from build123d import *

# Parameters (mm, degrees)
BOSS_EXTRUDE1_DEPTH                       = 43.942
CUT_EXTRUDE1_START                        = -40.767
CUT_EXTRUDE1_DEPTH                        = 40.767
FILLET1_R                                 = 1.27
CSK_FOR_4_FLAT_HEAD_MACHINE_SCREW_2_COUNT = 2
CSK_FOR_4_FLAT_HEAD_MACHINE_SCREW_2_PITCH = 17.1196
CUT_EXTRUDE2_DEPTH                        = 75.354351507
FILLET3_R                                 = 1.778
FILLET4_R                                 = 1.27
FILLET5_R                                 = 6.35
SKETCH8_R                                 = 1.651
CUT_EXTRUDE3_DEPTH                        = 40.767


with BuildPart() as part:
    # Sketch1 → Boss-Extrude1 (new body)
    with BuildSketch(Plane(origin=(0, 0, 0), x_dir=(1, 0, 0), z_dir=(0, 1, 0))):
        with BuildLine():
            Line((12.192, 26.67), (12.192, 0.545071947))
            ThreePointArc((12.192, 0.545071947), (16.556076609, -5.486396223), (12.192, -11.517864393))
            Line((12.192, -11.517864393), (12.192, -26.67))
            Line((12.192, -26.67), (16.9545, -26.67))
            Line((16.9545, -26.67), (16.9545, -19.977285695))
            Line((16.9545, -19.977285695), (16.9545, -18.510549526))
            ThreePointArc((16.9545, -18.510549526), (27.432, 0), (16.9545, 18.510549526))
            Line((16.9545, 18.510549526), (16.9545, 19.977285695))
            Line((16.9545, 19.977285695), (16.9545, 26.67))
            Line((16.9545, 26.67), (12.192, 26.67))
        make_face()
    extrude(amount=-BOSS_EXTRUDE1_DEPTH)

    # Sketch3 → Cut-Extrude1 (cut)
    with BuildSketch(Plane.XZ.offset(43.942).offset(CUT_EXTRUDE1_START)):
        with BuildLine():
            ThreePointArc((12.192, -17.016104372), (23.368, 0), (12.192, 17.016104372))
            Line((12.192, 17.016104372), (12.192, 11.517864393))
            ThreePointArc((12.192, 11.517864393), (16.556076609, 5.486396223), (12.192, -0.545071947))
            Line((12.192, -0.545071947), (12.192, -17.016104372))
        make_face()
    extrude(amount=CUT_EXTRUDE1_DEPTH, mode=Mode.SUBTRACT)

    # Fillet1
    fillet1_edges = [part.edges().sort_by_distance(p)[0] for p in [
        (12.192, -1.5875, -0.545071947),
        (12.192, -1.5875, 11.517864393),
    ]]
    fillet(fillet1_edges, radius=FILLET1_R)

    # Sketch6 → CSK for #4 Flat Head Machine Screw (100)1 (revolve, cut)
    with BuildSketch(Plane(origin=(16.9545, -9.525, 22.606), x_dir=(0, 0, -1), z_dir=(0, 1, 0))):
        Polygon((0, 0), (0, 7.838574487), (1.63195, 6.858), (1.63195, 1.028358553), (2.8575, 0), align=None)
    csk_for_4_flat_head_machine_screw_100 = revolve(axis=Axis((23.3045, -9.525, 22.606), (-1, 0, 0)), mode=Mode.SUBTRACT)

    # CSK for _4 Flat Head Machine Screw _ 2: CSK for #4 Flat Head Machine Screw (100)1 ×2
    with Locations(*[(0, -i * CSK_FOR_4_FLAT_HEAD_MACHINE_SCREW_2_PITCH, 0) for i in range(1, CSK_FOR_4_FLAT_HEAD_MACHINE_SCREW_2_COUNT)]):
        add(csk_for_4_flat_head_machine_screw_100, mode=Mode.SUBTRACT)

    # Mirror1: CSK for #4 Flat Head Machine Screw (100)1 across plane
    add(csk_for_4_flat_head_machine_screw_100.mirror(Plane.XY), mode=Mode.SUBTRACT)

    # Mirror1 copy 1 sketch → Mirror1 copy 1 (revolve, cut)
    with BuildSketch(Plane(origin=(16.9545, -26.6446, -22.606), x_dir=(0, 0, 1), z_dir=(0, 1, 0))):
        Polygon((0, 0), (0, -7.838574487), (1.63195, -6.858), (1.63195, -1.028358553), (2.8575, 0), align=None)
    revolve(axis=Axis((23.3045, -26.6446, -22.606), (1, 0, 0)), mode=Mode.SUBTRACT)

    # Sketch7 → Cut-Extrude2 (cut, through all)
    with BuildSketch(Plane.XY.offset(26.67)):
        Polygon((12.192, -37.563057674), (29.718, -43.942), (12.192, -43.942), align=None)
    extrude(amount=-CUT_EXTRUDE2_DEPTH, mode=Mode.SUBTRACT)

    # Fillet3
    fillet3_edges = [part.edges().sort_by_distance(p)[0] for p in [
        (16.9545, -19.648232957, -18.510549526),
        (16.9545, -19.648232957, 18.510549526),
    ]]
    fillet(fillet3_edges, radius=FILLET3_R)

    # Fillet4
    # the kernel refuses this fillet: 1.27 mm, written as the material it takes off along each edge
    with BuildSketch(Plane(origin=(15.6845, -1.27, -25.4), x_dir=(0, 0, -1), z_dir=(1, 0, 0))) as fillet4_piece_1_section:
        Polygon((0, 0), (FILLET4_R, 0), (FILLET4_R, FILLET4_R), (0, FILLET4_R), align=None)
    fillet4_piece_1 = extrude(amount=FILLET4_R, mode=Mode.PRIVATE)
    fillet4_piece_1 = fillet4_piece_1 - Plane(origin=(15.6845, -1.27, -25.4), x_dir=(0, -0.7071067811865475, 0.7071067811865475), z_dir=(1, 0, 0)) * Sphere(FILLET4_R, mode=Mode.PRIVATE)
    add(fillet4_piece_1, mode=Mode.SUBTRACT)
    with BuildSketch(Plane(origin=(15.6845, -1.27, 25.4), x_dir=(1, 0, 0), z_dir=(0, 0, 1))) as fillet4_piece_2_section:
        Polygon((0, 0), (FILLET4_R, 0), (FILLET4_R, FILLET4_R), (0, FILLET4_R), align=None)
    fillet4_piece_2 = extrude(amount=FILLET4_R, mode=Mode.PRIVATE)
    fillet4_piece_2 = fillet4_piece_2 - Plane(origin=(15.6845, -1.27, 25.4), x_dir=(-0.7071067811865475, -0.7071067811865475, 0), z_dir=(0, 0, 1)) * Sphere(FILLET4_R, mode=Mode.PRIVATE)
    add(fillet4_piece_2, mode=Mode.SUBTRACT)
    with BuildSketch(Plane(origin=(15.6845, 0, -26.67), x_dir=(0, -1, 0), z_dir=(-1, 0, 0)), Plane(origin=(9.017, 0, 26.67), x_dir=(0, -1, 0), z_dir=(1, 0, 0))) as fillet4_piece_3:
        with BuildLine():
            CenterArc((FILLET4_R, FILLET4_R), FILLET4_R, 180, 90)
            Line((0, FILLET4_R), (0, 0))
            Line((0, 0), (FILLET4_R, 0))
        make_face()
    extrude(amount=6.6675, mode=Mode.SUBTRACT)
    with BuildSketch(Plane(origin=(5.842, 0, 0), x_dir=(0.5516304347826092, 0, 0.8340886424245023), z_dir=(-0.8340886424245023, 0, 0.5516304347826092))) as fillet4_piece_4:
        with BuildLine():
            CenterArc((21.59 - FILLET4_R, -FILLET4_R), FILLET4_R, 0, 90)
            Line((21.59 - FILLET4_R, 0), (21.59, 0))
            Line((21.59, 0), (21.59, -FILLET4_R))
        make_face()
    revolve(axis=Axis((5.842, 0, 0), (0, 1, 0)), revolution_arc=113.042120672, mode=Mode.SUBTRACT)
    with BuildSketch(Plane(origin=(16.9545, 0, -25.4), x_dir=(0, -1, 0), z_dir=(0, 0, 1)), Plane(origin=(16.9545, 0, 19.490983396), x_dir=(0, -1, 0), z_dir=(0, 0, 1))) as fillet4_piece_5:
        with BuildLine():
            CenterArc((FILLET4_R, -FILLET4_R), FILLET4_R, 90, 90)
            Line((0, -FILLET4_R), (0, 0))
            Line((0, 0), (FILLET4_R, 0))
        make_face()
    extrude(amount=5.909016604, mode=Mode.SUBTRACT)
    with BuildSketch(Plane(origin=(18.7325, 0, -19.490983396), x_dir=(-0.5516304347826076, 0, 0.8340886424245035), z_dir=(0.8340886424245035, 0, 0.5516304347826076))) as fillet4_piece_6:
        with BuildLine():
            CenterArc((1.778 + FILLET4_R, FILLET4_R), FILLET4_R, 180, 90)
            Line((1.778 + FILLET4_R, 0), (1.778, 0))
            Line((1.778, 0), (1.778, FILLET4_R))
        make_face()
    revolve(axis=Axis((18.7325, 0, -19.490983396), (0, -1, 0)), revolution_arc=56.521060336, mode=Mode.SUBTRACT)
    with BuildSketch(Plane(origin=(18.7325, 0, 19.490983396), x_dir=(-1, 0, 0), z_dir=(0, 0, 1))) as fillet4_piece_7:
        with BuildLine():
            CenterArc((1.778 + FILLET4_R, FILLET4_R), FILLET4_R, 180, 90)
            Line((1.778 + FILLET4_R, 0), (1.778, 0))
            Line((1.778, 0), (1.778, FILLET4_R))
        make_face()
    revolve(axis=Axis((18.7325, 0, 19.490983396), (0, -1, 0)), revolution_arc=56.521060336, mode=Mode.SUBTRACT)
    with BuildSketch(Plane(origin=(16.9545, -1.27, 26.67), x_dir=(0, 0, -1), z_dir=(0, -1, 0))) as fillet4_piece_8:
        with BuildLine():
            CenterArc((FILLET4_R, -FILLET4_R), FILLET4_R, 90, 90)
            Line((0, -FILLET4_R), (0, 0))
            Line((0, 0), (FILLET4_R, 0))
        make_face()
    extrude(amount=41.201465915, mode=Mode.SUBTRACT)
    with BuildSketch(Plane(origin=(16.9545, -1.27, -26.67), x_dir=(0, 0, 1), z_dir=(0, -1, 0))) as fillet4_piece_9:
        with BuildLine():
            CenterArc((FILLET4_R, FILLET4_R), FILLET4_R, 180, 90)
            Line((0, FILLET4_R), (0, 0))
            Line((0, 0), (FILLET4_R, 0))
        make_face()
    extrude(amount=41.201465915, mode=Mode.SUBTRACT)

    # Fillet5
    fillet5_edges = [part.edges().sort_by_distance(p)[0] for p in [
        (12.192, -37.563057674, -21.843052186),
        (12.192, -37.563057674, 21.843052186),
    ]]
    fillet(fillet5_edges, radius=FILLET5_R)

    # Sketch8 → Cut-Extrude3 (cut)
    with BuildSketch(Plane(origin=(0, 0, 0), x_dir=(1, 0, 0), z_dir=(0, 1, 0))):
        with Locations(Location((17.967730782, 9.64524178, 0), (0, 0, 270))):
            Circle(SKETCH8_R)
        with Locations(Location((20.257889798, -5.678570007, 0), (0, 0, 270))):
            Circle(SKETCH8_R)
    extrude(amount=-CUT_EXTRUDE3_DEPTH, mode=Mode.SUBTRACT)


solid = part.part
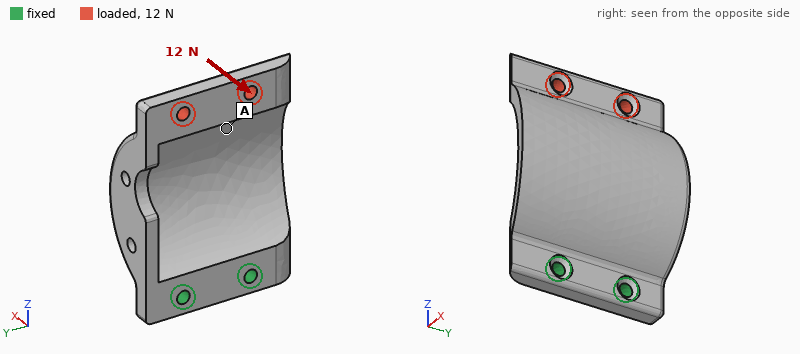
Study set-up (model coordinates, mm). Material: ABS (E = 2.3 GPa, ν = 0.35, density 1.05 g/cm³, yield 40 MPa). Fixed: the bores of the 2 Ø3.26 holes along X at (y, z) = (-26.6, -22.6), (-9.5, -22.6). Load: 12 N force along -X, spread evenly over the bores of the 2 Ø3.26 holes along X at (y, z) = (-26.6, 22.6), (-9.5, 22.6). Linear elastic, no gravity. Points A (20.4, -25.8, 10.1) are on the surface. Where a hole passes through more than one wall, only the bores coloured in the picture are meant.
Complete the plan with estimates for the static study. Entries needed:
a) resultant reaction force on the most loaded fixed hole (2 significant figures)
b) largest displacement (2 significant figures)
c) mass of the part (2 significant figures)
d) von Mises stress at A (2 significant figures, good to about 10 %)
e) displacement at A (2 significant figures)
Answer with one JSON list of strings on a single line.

["8.5 N", "0.70 mm", "11 g", "0.79 MPa", "0.38 mm"]
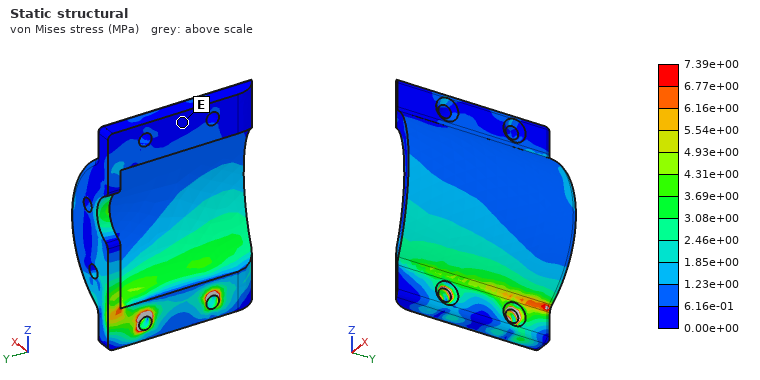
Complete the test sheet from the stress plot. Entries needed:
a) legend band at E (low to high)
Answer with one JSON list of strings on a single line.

["0.00e+00 to 6.16e-01 MPa"]
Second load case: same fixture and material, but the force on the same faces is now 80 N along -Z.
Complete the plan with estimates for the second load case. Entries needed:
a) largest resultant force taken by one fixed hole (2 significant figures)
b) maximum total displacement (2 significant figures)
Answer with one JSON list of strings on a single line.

["41 N", "0.77 mm"]
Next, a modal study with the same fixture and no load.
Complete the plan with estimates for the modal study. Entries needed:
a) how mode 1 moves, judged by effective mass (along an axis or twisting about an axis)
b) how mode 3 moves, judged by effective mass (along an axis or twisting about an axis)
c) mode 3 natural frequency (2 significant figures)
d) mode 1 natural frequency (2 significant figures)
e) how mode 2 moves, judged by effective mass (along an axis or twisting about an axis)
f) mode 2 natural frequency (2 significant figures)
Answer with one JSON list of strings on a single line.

["along X", "along Z", "1500 Hz", "380 Hz", "along Y", "690 Hz"]
